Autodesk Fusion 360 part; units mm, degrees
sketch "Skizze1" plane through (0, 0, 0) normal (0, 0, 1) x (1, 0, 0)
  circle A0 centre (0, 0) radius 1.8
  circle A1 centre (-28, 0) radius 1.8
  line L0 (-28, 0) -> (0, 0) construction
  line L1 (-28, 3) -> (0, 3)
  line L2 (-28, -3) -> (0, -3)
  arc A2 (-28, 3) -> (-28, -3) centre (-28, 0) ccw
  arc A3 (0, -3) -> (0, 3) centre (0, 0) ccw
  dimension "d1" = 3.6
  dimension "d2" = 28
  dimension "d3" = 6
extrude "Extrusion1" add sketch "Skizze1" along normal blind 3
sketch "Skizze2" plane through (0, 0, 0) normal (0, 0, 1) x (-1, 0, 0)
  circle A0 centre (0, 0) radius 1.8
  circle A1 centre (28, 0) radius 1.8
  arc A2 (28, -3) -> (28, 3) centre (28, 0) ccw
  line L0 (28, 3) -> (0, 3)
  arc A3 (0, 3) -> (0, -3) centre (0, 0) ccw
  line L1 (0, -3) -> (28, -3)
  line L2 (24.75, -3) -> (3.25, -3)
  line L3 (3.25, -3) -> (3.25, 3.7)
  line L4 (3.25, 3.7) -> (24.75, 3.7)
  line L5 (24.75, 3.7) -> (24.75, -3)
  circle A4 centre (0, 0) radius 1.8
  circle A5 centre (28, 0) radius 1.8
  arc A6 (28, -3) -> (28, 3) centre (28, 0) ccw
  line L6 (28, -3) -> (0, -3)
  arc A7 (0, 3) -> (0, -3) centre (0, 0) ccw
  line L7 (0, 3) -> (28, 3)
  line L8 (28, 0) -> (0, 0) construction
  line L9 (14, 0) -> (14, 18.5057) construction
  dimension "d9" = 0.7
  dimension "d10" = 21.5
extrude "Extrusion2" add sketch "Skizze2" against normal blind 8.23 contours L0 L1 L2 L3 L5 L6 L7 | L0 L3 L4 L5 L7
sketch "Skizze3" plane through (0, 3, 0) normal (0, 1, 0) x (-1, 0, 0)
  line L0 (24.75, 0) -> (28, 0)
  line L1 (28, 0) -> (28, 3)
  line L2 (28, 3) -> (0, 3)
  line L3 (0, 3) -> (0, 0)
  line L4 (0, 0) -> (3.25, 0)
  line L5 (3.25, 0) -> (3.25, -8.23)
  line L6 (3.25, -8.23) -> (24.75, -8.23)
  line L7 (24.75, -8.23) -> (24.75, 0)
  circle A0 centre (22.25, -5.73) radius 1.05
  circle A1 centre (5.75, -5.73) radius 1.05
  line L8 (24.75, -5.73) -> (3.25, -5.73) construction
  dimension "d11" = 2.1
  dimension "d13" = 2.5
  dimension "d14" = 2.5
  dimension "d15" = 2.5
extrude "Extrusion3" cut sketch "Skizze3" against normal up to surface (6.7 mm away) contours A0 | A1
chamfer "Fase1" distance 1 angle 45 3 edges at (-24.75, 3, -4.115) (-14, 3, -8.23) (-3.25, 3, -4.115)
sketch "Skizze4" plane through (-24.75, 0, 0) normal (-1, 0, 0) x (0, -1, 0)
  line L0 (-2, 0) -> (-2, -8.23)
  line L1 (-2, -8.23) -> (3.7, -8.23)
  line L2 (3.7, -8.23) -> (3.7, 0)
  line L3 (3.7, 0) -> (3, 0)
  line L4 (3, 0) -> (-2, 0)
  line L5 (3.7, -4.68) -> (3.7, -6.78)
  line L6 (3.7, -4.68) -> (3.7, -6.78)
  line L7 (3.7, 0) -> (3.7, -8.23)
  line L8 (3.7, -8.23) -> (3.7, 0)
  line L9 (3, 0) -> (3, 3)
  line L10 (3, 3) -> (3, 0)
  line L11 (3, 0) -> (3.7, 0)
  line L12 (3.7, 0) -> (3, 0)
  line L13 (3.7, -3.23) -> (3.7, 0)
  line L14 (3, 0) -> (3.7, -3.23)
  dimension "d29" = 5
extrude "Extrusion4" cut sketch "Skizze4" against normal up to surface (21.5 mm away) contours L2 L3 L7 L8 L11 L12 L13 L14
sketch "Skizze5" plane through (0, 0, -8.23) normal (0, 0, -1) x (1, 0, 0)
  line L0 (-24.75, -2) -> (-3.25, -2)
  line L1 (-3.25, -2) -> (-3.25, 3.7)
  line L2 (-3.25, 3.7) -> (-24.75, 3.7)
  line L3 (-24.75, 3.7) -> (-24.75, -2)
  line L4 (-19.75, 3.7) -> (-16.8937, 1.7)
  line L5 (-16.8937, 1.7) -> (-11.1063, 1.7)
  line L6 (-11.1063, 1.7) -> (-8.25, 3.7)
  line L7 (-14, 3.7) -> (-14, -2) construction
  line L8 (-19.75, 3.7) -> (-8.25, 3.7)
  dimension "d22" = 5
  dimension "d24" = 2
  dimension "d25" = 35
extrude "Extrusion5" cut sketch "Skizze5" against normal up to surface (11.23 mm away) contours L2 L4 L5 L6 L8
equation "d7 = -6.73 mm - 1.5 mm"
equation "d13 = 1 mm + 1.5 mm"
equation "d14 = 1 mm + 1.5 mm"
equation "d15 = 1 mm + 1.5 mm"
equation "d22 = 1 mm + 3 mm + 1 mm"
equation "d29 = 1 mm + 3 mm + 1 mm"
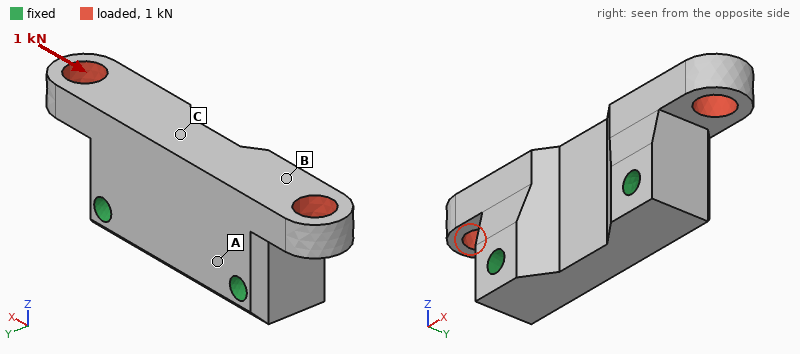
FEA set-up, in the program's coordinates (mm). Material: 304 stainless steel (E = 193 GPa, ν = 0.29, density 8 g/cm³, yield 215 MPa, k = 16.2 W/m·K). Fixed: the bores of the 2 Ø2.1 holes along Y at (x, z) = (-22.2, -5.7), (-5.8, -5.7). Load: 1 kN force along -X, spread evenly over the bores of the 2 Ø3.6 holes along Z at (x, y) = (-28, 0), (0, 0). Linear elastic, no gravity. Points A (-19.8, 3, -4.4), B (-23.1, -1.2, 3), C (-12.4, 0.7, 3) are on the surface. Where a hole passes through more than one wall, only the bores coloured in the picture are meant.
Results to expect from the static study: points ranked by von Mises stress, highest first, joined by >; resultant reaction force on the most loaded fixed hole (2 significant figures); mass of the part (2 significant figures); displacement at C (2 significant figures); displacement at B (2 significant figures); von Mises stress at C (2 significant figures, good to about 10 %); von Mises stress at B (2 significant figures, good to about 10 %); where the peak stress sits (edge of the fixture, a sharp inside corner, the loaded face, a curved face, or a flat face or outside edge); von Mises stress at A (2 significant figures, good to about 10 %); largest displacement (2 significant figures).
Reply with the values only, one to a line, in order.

B > A > C
620 N
12 g
0.98 µm
1.9 µm
8.2 MPa
30 MPa
the loaded face
18 MPa
5.0 µm
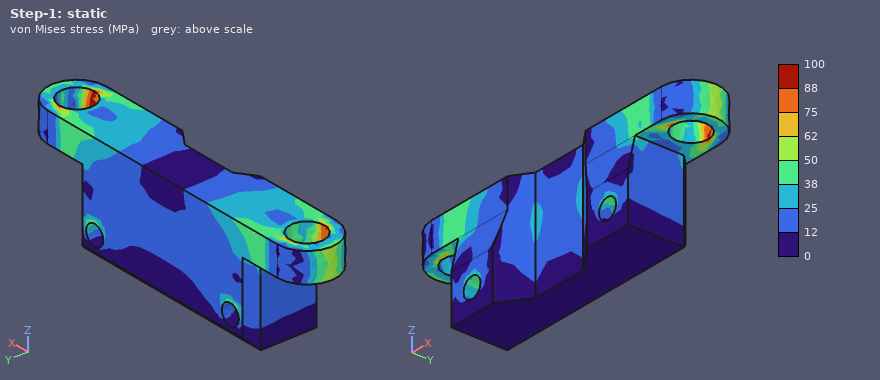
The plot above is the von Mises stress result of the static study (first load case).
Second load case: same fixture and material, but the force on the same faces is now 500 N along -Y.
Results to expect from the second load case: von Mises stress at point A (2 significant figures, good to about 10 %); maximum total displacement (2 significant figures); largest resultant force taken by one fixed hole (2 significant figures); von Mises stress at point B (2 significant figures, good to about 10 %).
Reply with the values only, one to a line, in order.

16 MPa
11 µm
250 N
15 MPa
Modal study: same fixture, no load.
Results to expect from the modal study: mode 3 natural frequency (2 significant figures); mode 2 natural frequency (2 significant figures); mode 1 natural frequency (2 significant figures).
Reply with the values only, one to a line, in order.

40 kHz
36 kHz
36 kHz
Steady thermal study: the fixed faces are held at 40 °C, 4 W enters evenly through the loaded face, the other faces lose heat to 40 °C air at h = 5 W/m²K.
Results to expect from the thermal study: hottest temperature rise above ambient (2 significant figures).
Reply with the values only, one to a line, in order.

72 K
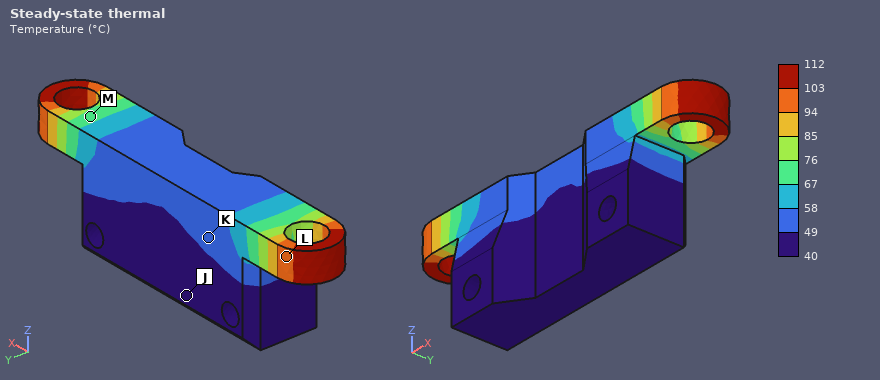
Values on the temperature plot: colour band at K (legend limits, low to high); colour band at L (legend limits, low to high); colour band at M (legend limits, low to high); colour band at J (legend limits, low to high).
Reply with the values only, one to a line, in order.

49 to 58 °C
94 to 103 °C
67 to 76 °C
40 to 49 °C
